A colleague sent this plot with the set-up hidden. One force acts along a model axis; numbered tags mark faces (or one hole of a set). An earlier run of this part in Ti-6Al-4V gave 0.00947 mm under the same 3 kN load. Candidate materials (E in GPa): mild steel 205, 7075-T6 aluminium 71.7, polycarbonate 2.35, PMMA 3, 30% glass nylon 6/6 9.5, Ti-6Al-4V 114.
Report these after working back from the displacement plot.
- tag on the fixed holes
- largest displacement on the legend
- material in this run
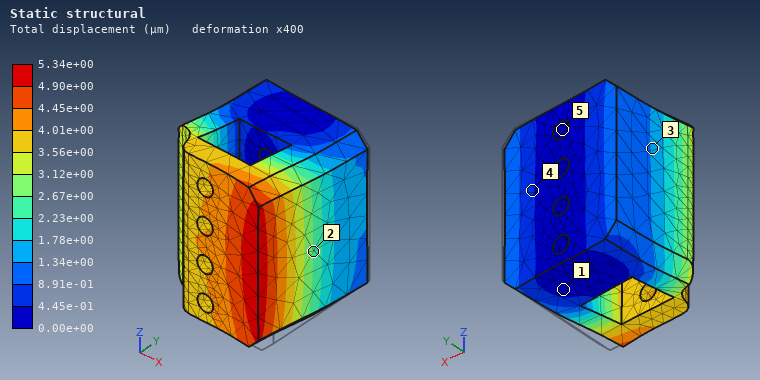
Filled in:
5
5.34e+00 µm
mild steel
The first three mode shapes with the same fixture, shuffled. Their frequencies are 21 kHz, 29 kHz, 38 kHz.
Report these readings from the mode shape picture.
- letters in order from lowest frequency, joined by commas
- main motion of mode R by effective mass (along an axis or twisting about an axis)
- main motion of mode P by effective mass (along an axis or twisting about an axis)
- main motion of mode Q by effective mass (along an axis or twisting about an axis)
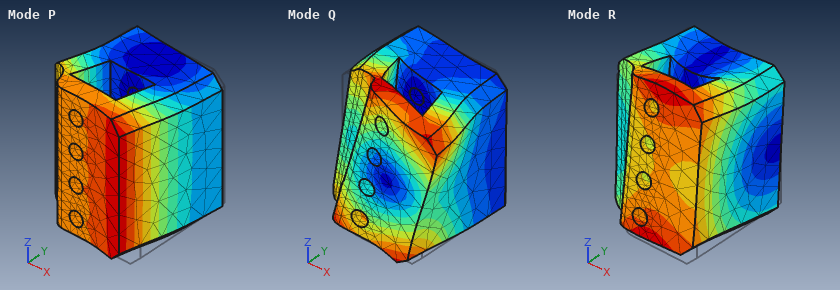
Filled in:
P, R, Q
along Z
along X
twisting about Y
